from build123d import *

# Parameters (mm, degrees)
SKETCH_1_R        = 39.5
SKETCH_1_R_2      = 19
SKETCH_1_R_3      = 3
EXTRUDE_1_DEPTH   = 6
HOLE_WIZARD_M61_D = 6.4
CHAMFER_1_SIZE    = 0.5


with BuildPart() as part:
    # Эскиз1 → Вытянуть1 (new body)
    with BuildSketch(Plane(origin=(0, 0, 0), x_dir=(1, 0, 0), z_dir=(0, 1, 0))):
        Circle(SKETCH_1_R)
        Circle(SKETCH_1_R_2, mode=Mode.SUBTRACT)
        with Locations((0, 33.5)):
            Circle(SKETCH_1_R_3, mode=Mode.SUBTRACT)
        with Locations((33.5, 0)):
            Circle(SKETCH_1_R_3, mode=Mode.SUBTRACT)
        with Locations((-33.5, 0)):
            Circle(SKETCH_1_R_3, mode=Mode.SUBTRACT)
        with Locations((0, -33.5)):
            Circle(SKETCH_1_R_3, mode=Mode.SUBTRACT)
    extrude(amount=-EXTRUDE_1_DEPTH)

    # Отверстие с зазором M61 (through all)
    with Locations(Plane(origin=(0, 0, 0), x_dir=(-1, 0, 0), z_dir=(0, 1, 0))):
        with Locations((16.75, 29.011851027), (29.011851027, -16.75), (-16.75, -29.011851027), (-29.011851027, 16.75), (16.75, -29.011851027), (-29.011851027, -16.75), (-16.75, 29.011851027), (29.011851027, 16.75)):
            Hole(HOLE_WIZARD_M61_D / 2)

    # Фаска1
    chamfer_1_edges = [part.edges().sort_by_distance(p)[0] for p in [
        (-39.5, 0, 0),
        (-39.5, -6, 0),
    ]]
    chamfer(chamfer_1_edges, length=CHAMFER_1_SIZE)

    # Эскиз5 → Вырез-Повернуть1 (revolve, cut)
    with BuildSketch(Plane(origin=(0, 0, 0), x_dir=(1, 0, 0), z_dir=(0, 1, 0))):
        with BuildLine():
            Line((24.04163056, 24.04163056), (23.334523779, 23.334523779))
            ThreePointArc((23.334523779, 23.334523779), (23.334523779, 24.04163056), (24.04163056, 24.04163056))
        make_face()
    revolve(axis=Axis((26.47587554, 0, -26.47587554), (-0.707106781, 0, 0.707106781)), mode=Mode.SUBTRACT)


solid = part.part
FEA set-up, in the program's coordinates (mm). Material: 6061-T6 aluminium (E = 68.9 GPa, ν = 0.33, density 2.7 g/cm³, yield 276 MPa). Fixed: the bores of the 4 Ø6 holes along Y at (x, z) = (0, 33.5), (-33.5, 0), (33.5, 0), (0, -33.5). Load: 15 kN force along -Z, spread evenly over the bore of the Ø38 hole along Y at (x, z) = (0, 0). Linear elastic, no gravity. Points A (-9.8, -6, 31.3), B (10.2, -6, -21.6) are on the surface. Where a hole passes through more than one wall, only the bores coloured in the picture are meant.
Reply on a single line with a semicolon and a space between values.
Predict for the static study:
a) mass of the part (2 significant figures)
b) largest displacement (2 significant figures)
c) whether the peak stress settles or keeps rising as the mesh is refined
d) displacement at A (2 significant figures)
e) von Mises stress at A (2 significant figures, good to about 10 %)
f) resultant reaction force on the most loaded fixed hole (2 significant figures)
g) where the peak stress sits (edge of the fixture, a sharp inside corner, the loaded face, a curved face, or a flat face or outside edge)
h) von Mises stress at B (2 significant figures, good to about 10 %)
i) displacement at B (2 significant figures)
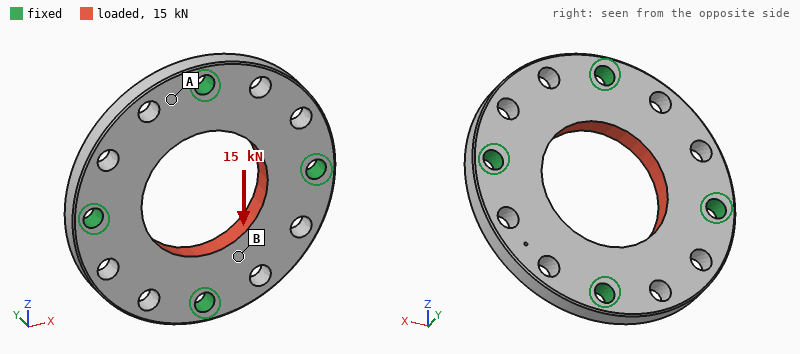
55 g; 16 µm; keeps rising; 6.6 µm; 20 MPa; 4.1 kN; edge of the fixture; 38 MPa; 11 µm
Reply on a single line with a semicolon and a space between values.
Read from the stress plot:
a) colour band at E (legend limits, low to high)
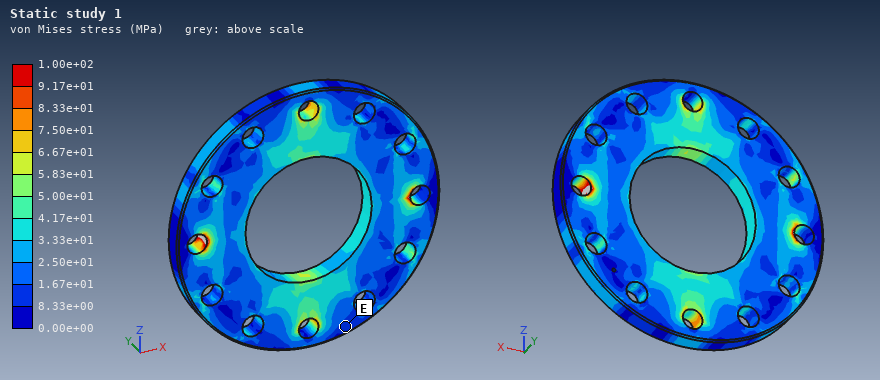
8.33e+00 to 1.67e+01 MPa
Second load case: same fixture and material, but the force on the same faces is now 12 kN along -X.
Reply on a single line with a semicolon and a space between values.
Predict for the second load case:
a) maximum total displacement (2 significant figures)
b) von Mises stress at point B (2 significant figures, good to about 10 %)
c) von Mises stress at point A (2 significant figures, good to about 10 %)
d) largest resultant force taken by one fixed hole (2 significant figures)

13 µm; 11 MPa; 11 MPa; 3.3 kN
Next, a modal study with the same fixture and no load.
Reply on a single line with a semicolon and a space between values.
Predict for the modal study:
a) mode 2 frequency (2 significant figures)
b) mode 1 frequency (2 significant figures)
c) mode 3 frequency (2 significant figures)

12 kHz; 11 kHz; 12 kHz
